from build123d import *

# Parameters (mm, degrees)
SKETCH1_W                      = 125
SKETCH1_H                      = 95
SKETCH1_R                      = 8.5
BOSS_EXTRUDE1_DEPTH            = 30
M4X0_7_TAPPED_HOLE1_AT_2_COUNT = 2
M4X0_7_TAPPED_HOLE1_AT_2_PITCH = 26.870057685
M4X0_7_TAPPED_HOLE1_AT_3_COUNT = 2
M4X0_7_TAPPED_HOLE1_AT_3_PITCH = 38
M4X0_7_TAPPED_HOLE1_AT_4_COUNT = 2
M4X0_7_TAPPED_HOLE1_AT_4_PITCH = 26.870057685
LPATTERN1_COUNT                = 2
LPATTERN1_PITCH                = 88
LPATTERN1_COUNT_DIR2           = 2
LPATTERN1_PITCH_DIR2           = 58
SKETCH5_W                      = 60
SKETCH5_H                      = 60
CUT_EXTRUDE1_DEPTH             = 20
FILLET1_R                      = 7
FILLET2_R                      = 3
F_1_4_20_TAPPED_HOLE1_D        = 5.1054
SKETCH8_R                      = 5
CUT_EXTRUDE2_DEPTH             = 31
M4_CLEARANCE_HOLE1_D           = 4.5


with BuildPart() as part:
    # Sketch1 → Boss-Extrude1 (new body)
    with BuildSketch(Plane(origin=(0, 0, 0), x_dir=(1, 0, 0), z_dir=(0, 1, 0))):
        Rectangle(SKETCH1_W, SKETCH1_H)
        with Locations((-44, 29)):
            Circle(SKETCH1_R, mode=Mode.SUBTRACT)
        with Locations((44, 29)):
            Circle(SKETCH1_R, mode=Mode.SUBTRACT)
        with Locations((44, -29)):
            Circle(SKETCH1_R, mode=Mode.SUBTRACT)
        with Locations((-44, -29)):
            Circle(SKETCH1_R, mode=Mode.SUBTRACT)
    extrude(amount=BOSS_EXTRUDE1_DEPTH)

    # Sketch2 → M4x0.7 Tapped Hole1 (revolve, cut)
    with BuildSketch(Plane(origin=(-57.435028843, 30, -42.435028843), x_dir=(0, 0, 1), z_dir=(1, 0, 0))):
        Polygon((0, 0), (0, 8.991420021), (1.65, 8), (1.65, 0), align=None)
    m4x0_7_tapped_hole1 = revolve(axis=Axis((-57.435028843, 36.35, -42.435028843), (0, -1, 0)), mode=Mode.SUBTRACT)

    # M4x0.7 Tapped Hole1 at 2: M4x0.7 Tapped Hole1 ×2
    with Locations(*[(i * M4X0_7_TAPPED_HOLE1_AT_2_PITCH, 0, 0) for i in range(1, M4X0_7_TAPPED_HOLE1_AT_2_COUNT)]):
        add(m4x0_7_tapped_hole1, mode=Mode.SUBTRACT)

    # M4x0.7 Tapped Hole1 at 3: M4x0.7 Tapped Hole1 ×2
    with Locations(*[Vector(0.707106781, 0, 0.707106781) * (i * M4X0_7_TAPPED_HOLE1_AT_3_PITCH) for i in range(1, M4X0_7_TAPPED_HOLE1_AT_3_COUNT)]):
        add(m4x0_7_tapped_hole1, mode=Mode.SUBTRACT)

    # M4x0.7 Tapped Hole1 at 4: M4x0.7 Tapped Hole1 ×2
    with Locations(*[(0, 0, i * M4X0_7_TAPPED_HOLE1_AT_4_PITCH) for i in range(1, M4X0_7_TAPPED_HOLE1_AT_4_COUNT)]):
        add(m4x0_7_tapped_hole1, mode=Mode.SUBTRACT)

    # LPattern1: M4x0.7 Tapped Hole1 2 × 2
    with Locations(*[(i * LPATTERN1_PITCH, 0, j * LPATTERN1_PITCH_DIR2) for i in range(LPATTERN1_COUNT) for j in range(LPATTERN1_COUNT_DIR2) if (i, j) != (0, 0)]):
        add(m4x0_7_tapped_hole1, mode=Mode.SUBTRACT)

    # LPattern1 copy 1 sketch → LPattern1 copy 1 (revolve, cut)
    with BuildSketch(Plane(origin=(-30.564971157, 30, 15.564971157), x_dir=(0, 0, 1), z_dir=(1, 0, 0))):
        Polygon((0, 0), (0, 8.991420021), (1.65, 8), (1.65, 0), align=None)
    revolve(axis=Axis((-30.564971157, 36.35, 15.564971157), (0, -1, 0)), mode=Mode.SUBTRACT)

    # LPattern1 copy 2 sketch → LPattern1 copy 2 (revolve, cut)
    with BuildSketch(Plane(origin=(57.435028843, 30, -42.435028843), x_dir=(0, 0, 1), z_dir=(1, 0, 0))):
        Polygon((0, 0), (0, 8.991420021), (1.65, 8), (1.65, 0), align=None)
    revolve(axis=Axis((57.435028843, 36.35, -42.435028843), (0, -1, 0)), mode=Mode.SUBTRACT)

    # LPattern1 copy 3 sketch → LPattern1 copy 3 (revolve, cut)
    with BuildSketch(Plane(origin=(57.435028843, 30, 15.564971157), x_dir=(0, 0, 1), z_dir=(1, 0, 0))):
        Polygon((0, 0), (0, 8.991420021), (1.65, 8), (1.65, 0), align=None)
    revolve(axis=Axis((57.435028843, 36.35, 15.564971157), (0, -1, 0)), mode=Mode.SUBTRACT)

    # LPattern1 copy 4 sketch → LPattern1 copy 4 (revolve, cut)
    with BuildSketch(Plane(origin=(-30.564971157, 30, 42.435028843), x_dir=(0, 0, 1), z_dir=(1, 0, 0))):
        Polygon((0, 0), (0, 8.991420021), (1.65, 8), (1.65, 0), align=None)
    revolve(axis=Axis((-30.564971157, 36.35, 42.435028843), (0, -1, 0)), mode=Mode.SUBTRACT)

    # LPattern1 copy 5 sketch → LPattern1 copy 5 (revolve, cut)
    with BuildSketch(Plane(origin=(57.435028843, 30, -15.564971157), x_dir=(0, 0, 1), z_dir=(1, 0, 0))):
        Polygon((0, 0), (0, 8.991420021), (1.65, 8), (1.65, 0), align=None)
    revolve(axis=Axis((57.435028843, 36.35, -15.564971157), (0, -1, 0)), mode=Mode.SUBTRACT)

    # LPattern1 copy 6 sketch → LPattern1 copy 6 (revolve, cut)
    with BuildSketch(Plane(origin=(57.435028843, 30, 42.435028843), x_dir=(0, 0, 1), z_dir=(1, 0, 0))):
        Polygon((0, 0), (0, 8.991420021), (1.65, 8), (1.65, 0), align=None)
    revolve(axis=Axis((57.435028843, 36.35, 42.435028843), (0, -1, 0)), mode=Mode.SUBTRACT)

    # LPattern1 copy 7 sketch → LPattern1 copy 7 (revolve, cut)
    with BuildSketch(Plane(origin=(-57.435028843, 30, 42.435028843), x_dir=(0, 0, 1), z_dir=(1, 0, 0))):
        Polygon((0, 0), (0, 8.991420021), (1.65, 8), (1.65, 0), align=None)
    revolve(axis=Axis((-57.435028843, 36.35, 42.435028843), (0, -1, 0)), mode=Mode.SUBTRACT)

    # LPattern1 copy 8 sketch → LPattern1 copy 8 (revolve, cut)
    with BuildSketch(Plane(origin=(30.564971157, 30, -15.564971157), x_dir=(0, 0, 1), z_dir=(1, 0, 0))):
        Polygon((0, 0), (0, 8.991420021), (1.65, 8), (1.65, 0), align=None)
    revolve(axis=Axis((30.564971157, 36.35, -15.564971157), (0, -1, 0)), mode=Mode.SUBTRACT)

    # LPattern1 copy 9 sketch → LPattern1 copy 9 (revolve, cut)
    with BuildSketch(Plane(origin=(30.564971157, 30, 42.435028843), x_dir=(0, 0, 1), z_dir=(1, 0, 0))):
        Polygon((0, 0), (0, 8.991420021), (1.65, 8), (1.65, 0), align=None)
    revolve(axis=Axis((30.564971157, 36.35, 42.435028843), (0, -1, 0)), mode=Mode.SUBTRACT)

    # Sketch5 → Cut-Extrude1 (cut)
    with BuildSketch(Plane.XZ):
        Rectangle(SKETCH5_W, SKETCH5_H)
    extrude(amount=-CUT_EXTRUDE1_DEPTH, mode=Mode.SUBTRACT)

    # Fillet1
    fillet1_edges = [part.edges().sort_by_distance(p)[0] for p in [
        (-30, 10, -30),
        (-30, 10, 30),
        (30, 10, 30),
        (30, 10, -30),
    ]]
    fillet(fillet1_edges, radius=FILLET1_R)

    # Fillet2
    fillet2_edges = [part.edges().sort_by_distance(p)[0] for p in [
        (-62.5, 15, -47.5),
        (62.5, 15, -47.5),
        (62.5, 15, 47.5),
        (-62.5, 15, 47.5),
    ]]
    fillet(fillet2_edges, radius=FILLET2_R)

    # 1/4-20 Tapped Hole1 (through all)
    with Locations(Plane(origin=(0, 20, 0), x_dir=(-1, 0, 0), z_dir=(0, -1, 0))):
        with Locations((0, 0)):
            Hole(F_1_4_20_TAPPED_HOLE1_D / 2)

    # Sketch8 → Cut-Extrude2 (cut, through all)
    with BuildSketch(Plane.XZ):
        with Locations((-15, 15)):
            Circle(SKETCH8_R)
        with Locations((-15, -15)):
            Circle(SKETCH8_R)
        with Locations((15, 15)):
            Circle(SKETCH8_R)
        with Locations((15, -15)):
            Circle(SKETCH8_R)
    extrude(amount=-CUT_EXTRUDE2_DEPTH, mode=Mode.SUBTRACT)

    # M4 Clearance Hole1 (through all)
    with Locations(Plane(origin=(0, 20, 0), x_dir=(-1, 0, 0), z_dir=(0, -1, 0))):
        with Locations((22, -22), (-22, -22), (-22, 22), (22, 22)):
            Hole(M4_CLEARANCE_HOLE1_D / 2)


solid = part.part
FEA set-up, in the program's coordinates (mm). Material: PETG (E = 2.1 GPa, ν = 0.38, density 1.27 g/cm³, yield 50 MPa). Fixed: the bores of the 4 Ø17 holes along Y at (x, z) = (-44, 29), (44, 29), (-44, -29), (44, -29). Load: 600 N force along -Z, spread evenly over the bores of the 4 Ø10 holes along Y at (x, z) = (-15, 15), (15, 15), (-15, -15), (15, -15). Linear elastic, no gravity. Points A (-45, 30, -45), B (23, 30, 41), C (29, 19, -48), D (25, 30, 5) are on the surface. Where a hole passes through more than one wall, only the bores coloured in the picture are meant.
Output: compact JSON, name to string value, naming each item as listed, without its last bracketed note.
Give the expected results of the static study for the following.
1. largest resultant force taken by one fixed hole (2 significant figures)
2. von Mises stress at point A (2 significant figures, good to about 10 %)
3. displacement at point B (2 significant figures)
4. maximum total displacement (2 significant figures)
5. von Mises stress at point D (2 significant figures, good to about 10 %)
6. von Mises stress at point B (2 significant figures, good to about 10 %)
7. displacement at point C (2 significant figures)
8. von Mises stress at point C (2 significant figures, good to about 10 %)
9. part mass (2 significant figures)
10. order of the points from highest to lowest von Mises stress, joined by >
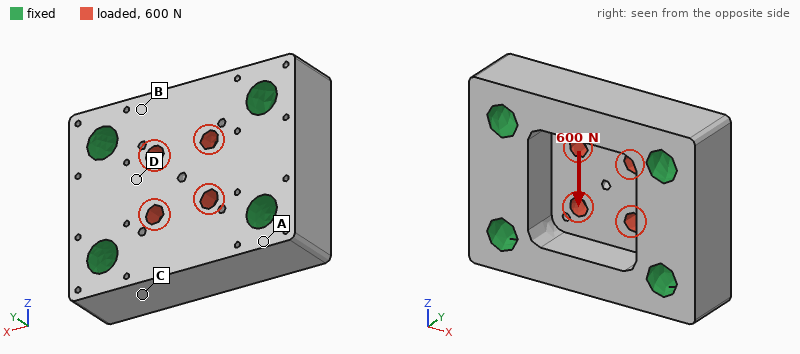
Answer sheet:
{"largest resultant force taken by one fixed hole": "160 N", "von Mises stress at point A": "0.10 MPa", "displacement at point B": "6.4 µm", "maximum total displacement": "13 µm", "von Mises stress at point D": "0.50 MPa", "von Mises stress at point B": "0.39 MPa", "displacement at point C": "3.7 µm", "von Mises stress at point C": "0.23 MPa", "part mass": "320 g", "order of the points from highest to lowest von Mises stress, joined by >": "D > B > C > A"}
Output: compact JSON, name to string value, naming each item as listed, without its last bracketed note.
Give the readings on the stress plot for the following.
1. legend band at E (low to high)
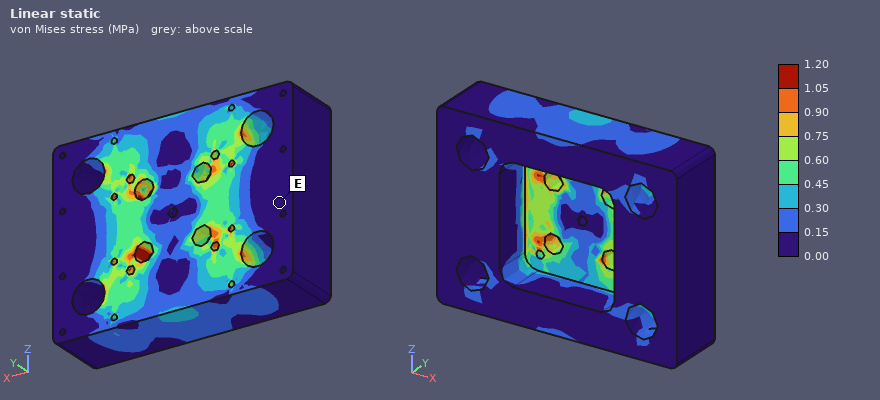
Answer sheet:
{"legend band at E": "0.00 to 0.15 MPa"}
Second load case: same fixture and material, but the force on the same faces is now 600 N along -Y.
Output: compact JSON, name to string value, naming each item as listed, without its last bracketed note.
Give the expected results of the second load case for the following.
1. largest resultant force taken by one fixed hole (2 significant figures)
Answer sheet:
{"largest resultant force taken by one fixed hole": "160 N"}
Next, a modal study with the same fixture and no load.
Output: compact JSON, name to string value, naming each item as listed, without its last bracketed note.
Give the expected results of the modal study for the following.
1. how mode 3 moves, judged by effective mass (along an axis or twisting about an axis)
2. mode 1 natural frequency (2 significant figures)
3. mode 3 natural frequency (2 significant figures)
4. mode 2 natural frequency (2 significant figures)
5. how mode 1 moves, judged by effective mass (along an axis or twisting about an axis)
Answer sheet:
{"how mode 3 moves, judged by effective mass": "along Z", "mode 1 natural frequency": "3200 Hz", "mode 3 natural frequency": "4000 Hz", "mode 2 natural frequency": "3800 Hz", "how mode 1 moves, judged by effective mass": "along Y"}
